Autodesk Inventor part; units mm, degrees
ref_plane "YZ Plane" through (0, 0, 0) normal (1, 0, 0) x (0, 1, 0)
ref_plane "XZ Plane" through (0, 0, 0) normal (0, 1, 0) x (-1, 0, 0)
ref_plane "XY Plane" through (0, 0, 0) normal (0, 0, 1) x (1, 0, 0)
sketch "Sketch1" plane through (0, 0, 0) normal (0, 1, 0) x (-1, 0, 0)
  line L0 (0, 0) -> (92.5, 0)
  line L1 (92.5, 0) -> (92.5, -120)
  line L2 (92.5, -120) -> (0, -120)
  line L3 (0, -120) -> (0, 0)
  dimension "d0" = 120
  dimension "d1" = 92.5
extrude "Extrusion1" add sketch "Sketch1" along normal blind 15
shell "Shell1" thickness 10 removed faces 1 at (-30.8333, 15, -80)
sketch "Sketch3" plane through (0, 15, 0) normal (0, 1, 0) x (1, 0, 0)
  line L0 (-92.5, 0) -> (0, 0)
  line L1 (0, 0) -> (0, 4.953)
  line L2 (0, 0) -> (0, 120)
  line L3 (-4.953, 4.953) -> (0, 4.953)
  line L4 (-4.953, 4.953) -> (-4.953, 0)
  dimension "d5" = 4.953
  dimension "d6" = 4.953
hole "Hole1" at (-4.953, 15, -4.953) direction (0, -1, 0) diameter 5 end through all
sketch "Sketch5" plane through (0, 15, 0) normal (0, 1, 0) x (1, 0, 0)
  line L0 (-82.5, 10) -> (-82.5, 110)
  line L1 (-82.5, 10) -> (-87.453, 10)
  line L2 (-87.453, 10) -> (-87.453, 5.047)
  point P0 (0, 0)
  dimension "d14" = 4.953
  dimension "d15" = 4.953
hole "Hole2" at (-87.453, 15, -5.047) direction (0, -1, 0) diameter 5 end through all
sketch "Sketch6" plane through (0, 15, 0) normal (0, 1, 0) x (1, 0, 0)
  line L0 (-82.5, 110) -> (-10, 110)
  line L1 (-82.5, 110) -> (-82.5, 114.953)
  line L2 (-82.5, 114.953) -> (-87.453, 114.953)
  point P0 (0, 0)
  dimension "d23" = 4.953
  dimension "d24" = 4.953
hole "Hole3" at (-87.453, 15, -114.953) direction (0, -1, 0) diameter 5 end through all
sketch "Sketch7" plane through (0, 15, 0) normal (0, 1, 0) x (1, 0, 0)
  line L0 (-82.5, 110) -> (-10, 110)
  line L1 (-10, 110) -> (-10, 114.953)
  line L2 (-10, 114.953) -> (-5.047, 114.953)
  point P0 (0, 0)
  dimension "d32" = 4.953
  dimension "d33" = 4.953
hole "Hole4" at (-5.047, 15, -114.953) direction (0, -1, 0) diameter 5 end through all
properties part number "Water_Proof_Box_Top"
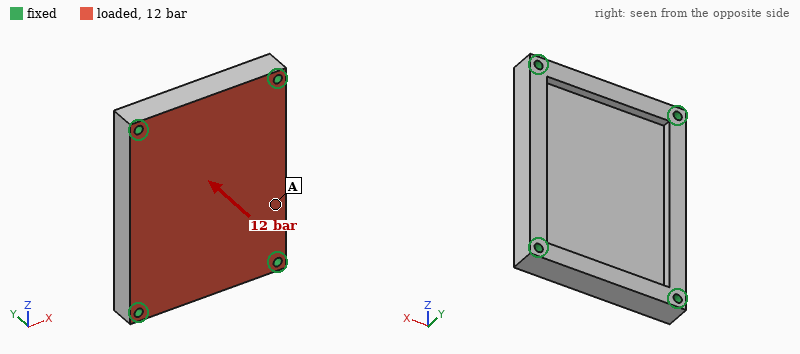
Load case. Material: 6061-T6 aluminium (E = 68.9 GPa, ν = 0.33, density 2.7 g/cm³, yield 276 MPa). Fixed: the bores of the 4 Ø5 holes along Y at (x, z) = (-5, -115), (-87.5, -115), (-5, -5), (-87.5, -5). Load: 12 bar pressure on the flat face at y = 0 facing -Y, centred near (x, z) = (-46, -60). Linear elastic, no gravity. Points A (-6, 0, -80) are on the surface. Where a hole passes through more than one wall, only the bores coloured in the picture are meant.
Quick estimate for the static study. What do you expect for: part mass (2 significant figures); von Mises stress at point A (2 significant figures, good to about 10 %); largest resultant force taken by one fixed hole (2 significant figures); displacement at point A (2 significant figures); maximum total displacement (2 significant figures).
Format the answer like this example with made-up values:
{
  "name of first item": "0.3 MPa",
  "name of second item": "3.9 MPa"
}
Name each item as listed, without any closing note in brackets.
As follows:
{
  "part mass": "350 g",
  "von Mises stress at point A": "22 MPa",
  "largest resultant force taken by one fixed hole": "3.5 kN",
  "displacement at point A": "0.056 mm",
  "maximum total displacement": "0.10 mm"
}
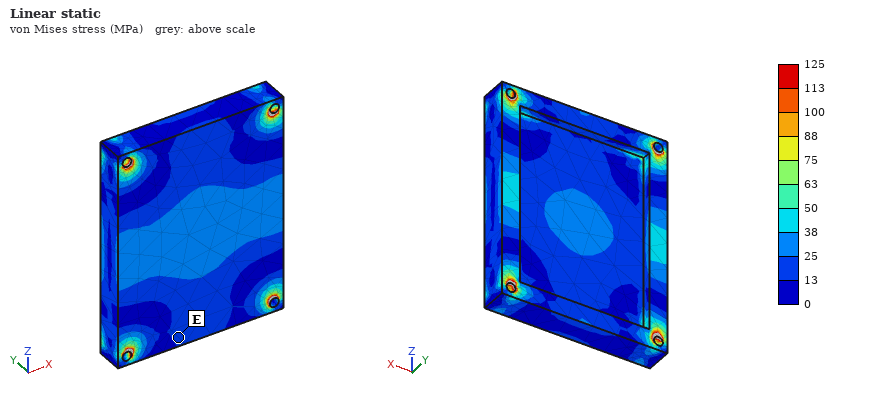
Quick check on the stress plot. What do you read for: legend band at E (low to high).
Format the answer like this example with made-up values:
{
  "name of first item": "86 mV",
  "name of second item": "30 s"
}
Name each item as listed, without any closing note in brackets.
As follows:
{
  "legend band at E": "13 to 25 MPa"
}
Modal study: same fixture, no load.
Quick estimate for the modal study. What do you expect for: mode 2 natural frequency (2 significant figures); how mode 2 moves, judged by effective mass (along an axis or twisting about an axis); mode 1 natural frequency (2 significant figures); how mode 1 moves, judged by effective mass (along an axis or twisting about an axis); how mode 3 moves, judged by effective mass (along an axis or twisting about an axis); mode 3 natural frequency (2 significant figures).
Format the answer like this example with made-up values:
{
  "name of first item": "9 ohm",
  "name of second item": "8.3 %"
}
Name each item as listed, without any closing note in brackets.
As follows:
{
  "mode 2 natural frequency": "5900 Hz",
  "how mode 2 moves, judged by effective mass": "twisting about Z",
  "mode 1 natural frequency": "3900 Hz",
  "how mode 1 moves, judged by effective mass": "along Y",
  "how mode 3 moves, judged by effective mass": "twisting about X",
  "mode 3 natural frequency": "8000 Hz"
}
